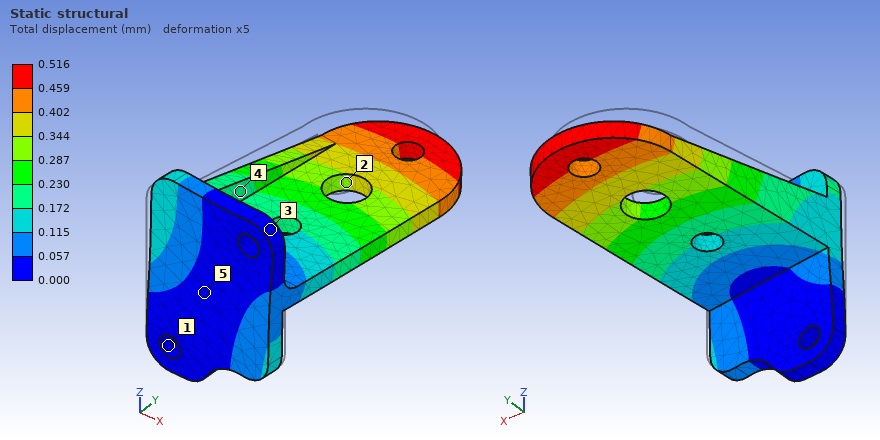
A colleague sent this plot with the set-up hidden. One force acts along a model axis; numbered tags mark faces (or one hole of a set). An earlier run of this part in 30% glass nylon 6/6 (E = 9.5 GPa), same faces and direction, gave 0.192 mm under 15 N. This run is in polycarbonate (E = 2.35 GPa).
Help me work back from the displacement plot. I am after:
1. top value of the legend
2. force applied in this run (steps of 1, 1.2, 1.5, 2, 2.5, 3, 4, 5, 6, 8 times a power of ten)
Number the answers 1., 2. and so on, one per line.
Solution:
1. 0.516 mm
2. 10 N
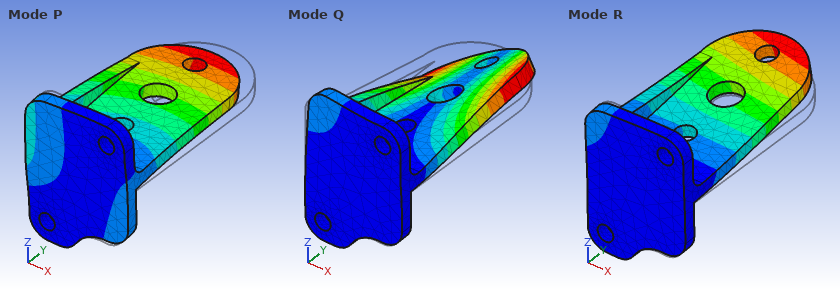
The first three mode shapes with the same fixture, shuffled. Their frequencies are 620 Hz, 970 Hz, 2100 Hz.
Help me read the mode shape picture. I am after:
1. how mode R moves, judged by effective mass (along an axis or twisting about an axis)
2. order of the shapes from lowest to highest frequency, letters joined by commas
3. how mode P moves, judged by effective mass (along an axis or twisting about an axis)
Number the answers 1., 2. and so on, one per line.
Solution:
1. along Z
2. R, P, Q
3. along X
